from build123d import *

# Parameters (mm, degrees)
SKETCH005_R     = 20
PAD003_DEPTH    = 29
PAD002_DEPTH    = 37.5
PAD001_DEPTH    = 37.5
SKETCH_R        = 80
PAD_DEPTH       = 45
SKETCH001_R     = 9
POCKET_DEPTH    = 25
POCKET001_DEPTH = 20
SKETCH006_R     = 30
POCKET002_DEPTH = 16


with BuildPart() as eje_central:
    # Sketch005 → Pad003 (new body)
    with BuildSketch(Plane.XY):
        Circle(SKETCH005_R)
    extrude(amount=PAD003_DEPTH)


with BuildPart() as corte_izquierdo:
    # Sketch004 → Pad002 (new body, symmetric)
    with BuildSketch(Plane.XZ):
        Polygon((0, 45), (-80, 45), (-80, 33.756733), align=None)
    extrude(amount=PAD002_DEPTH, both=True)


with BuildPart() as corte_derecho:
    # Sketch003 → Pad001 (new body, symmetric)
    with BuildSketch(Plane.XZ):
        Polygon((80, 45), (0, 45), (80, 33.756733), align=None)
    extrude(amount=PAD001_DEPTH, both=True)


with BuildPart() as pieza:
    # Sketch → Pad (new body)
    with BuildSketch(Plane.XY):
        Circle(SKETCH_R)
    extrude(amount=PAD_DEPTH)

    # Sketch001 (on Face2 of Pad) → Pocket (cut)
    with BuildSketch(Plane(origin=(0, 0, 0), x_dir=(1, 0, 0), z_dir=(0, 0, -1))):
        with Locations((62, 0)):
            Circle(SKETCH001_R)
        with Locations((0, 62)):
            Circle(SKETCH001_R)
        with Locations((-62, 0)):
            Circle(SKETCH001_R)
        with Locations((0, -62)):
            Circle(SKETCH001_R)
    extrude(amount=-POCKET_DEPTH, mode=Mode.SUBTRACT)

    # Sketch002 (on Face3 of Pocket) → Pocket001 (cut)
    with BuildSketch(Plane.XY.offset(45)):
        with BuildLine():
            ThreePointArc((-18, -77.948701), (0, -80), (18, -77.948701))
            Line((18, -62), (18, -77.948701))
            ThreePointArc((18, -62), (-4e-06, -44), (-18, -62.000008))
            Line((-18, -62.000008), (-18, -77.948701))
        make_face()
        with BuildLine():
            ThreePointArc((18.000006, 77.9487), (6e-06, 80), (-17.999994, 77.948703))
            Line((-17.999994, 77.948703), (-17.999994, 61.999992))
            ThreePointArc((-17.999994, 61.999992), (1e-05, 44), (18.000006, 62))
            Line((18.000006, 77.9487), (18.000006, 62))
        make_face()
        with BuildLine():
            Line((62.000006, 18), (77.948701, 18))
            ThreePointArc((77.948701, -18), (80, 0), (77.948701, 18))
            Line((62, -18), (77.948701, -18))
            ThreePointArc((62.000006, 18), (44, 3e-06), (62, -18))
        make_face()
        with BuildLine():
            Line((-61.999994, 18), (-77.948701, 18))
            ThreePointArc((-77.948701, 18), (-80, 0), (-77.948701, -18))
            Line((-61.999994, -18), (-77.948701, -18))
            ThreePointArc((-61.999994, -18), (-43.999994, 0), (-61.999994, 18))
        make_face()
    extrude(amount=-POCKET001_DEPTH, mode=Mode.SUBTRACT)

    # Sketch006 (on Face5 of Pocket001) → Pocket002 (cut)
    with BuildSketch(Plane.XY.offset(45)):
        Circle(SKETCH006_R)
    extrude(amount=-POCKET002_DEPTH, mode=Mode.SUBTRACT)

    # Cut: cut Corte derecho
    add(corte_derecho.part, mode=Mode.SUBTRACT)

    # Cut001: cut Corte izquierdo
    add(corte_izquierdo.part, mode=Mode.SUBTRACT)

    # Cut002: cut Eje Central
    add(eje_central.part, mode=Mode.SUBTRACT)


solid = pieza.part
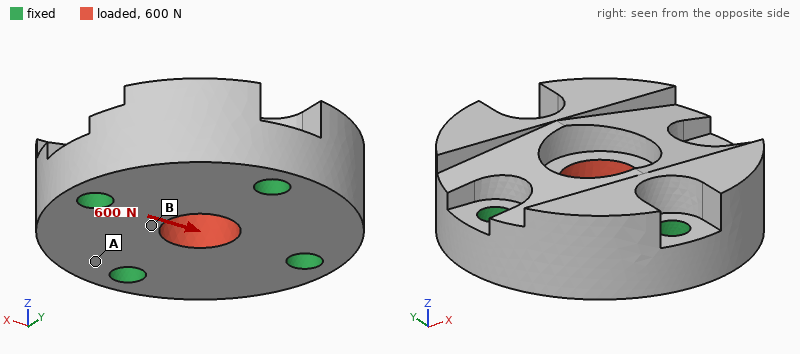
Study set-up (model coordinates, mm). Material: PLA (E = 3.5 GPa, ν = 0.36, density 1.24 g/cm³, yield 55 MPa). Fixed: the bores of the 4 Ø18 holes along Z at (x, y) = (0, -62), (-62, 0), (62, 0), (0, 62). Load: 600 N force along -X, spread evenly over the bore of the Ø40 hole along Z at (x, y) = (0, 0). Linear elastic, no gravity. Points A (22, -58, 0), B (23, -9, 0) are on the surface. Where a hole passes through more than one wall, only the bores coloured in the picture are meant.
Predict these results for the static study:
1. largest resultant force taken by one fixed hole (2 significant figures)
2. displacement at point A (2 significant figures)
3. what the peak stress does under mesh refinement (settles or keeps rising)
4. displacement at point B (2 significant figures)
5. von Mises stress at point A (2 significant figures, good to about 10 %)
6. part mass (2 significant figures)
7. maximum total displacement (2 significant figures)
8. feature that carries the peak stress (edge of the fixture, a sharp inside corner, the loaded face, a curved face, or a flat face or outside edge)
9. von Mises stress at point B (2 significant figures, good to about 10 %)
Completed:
190 N
0.42 µm
keeps rising
1.9 µm
0.063 MPa
830 g
2.4 µm
edge of the fixture
0.20 MPa
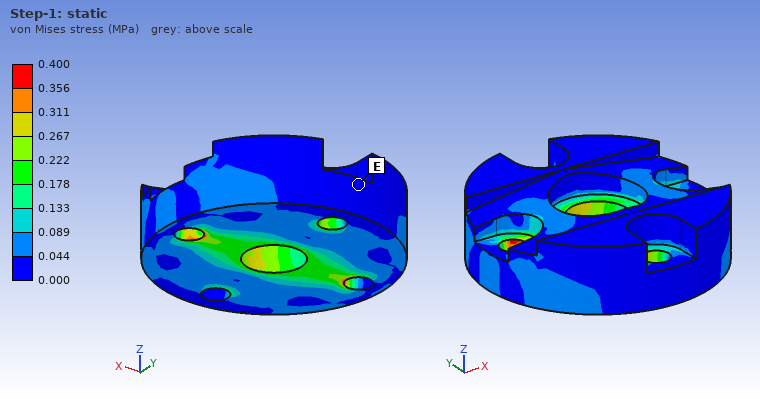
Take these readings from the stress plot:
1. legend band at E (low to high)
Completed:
0.000 to 0.044 MPa
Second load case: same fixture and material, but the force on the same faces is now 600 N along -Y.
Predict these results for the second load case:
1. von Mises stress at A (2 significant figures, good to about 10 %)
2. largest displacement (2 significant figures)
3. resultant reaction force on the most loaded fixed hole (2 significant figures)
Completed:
0.069 MPa
2.4 µm
190 N
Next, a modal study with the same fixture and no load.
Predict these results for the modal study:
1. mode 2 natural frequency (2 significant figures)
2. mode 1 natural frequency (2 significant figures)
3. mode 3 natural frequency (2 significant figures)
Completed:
3100 Hz
2900 Hz
3200 Hz
